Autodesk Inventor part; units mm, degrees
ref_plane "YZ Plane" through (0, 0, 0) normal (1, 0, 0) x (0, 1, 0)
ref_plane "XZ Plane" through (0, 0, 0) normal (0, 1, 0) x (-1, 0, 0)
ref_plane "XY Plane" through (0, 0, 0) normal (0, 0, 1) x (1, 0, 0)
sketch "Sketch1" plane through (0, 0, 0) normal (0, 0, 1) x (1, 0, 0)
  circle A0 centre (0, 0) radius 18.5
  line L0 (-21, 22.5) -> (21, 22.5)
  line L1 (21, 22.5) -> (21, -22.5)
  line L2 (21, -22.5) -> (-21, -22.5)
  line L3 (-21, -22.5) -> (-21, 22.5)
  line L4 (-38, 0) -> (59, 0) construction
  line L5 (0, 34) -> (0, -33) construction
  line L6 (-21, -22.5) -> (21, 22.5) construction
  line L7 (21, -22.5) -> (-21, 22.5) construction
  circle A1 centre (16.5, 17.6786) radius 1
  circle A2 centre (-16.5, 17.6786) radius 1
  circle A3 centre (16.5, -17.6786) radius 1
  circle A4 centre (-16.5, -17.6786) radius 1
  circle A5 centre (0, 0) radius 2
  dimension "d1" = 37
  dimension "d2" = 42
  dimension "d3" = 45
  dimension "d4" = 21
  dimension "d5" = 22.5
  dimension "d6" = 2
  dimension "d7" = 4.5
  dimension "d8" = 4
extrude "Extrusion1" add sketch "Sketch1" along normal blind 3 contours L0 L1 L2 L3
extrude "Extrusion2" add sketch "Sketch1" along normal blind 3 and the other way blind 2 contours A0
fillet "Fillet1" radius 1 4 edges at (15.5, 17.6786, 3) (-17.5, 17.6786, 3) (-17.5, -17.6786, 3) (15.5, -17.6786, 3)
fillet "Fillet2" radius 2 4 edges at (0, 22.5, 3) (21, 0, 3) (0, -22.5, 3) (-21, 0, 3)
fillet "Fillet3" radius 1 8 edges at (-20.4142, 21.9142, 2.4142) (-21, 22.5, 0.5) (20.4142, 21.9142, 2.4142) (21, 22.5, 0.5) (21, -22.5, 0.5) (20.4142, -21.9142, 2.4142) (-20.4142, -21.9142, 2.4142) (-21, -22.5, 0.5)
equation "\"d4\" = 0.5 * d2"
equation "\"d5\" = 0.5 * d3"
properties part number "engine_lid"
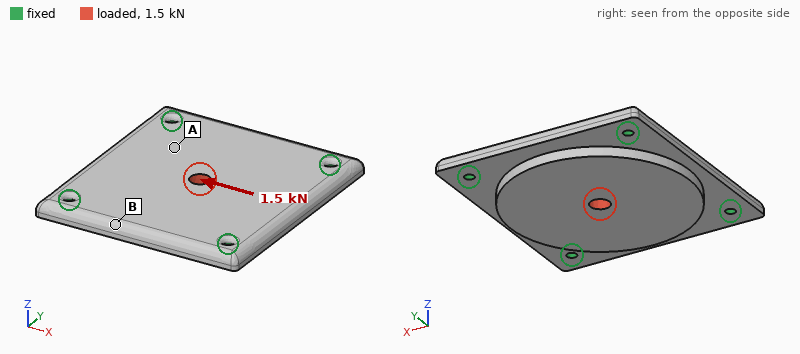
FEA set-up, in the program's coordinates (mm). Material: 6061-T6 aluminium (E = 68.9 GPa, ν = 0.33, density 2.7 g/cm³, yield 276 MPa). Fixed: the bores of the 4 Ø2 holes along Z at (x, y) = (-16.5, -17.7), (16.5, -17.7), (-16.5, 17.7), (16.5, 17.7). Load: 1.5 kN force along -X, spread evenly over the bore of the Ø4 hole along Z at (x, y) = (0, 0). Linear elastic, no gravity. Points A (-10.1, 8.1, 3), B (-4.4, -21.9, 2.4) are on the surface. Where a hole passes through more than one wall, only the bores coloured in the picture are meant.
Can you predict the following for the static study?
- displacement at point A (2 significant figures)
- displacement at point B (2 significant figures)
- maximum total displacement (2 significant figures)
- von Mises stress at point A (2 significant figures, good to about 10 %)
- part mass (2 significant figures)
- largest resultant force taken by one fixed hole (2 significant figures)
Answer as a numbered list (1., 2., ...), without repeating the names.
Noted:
1. 3.2 µm
2. 1.4 µm
3. 5.9 µm
4. 9.3 MPa
5. 20 g
6. 410 N
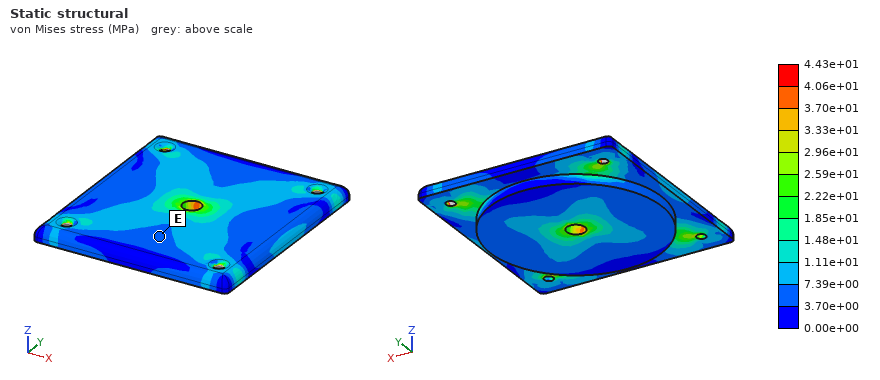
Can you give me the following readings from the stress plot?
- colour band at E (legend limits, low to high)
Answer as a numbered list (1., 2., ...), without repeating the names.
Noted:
1. 3.70e+00 to 7.39e+00 MPa
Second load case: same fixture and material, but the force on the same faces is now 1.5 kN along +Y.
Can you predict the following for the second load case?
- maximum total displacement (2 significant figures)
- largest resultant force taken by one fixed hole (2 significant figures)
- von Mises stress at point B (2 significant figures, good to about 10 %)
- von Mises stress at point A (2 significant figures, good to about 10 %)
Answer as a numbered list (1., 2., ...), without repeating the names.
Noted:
1. 5.5 µm
2. 400 N
3. 7.4 MPa
4. 9.4 MPa
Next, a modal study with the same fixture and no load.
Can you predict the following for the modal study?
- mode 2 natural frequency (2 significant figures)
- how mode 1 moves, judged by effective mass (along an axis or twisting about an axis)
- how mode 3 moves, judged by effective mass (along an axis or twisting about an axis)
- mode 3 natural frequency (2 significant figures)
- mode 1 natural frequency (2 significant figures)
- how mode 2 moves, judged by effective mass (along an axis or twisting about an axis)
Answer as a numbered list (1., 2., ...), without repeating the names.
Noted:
1. 14 kHz
2. along Z
3. twisting about X
4. 15 kHz
5. 8700 Hz
6. twisting about Y
